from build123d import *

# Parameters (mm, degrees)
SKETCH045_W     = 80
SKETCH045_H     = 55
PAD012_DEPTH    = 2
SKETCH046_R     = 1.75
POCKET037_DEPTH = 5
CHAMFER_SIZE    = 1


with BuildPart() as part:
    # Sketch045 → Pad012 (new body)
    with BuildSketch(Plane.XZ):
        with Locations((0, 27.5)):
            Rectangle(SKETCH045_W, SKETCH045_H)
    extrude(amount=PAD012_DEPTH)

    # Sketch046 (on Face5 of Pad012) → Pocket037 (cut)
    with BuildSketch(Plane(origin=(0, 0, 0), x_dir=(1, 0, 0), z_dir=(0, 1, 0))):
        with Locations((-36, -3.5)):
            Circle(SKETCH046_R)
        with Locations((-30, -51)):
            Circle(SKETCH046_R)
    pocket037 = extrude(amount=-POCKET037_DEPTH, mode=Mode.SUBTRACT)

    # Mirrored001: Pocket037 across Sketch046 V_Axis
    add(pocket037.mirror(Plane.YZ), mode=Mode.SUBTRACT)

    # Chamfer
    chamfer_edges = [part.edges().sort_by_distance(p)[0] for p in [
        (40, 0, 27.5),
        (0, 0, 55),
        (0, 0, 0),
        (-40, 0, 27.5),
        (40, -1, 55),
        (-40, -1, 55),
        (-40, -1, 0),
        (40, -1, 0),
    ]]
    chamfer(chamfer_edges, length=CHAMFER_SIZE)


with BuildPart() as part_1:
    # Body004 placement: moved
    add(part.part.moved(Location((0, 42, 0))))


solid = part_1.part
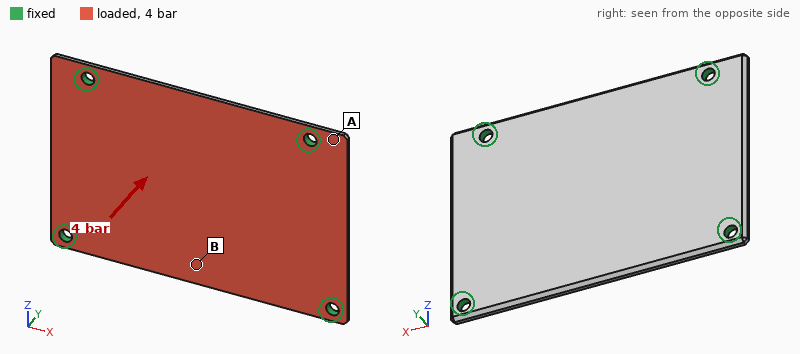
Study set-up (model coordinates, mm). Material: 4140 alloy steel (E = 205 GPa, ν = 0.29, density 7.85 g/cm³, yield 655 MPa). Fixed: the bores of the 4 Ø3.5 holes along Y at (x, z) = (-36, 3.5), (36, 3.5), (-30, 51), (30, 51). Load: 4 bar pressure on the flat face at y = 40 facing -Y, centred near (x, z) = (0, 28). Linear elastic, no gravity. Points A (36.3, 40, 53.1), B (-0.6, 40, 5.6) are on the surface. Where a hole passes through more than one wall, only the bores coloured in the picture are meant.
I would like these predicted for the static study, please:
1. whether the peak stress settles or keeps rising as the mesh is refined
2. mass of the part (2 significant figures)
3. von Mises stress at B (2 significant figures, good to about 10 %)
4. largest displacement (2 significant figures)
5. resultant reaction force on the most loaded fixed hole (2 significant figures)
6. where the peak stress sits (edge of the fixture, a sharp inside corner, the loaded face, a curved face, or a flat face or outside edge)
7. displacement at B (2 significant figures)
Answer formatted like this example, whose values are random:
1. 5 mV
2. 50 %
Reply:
1. keeps rising
2. 67 g
3. 140 MPa
4. 0.26 mm
5. 460 N
6. edge of the fixture
7. 0.26 mm
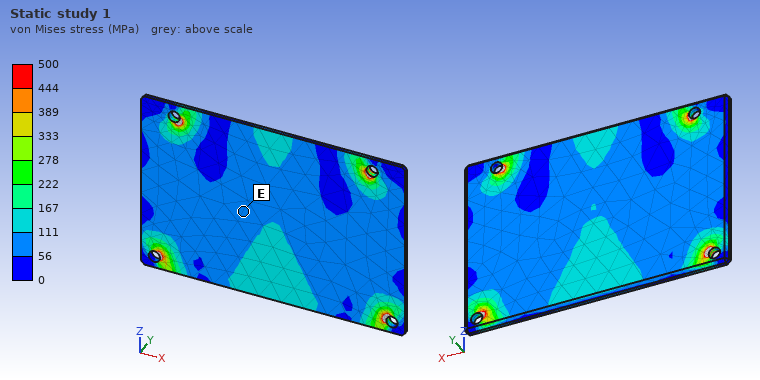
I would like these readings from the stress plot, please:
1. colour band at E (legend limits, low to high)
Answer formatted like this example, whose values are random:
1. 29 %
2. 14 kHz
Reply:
1. 56 to 111 MPa
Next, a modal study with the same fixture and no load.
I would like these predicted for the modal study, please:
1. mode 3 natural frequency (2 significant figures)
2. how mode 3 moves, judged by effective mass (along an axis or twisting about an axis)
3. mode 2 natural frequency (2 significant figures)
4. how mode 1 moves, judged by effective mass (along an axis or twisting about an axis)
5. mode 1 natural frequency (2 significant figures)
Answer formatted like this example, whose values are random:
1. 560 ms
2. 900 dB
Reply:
1. 4400 Hz
2. twisting about Z
3. 3300 Hz
4. along Y
5. 1900 Hz
